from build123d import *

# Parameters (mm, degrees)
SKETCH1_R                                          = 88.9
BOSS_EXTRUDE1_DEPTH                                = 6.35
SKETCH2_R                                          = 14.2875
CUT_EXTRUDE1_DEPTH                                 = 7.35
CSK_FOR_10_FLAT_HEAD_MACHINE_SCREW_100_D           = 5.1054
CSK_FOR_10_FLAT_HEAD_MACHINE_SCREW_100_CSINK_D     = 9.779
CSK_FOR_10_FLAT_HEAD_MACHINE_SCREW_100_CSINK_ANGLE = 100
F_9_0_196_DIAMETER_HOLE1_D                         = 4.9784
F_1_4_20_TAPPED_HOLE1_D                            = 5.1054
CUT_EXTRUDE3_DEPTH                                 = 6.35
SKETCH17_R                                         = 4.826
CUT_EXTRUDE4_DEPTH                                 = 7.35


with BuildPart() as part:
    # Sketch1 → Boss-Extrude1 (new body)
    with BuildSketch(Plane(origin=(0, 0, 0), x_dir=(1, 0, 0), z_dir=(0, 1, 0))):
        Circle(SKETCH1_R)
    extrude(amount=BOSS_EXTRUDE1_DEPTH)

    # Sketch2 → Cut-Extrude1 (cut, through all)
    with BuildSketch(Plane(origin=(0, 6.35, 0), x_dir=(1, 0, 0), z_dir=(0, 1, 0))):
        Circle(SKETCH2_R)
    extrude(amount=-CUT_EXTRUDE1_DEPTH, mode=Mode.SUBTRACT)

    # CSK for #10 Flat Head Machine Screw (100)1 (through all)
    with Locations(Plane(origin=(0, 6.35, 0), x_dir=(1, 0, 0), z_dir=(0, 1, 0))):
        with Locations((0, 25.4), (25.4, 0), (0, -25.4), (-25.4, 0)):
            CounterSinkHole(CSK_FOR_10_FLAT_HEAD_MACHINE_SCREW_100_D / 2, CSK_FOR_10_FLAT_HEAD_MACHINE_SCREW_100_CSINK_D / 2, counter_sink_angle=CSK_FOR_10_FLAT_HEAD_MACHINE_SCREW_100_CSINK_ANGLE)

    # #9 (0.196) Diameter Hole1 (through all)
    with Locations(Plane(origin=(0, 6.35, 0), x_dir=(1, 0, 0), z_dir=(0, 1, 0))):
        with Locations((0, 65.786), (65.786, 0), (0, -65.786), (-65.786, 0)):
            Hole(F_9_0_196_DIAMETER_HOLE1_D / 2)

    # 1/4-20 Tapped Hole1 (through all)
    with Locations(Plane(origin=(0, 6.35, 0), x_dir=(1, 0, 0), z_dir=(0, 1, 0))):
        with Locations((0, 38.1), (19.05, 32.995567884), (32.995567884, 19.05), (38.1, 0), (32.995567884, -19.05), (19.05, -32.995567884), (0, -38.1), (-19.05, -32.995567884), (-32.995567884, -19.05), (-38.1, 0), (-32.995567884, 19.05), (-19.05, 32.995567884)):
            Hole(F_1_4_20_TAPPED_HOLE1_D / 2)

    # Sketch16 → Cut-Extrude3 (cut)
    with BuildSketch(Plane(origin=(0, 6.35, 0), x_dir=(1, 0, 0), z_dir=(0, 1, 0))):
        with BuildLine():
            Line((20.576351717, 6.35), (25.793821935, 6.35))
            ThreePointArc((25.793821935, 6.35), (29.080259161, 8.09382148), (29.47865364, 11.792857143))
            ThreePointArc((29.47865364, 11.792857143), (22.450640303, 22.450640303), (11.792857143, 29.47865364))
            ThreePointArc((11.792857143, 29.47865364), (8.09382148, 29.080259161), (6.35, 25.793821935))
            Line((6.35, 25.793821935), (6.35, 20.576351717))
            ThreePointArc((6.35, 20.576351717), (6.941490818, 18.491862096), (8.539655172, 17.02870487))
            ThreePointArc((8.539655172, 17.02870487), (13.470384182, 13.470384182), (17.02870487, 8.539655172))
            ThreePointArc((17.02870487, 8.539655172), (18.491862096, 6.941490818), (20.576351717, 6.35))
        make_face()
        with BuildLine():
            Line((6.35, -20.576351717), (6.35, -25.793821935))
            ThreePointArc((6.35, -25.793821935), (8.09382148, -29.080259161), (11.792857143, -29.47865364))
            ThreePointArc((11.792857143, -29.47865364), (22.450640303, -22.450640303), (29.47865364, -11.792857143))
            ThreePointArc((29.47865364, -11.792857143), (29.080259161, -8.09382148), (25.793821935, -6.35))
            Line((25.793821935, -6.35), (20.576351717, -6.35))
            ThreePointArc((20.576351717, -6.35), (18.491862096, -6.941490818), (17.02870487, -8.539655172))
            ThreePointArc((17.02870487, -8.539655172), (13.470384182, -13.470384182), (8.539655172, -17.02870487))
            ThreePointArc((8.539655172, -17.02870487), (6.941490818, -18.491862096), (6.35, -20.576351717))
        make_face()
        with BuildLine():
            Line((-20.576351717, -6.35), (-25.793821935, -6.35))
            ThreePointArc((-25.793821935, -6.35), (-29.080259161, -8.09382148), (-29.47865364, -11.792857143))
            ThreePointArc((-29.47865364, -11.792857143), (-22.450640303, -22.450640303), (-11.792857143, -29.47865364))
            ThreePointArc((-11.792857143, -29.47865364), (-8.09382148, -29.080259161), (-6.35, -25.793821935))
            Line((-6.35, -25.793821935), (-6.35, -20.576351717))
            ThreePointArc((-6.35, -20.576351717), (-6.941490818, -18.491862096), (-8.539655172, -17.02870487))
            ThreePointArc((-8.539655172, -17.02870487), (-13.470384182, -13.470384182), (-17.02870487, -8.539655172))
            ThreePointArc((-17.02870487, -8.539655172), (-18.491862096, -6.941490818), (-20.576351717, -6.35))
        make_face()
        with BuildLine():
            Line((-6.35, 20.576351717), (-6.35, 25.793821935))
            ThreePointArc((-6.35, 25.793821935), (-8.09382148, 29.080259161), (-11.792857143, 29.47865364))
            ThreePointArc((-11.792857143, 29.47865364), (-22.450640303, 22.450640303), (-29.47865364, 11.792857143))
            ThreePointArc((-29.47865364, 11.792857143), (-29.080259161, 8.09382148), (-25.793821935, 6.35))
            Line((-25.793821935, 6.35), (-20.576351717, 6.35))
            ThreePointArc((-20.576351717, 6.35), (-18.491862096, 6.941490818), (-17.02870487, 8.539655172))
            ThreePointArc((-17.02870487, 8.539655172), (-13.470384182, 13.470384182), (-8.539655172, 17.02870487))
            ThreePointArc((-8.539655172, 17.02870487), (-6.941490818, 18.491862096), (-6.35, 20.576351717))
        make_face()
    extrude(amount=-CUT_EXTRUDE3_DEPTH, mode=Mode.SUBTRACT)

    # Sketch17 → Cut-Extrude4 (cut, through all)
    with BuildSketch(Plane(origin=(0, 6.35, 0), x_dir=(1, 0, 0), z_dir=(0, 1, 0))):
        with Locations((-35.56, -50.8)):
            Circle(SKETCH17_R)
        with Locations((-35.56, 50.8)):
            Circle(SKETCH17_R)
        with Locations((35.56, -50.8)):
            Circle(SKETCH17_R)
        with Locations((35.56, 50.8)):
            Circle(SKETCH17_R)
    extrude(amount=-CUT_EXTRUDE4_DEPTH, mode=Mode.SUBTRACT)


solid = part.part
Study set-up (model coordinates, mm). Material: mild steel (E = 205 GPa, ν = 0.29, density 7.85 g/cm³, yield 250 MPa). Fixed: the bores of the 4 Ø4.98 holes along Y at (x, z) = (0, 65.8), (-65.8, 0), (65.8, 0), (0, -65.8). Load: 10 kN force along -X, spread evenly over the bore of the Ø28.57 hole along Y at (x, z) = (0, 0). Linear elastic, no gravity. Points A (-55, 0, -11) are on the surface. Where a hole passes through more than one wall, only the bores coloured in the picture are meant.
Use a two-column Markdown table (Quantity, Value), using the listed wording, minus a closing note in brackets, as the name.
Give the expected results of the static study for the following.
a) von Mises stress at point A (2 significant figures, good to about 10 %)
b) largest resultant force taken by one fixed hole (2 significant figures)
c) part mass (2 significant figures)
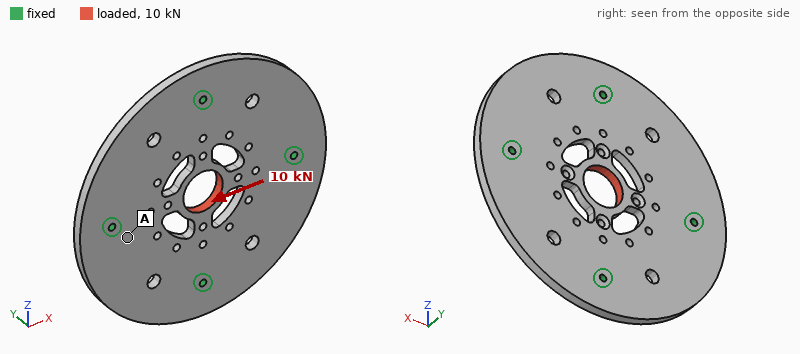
| Quantity | Value |
|---|---|
| von Mises stress at point A | 13 MPa |
| largest resultant force taken by one fixed hole | 3.2 kN |
| part mass | 1.1 kg |
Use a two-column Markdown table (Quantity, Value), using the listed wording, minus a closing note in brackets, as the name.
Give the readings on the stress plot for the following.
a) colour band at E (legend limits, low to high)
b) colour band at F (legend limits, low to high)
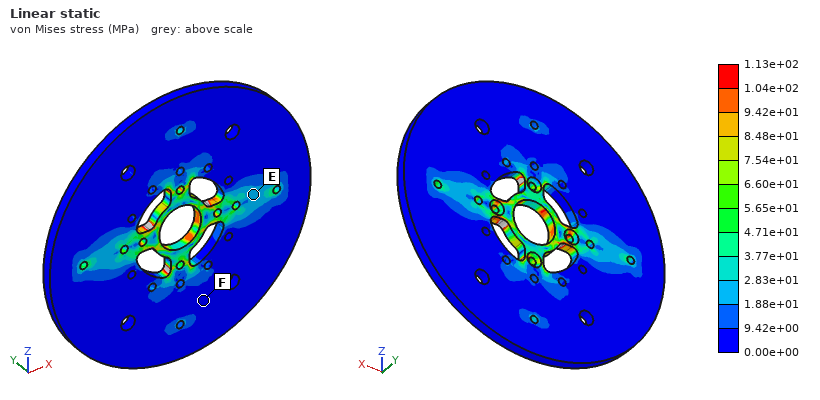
| Quantity | Value |
|---|---|
| colour band at E | 1.88e+01 to 2.83e+01 MPa |
| colour band at F | 0.00e+00 to 9.42e+00 MPa |
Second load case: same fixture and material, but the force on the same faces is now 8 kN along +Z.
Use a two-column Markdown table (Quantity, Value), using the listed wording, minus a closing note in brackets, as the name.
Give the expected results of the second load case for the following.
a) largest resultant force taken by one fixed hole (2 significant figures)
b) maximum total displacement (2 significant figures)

| Quantity | Value |
|---|---|
| largest resultant force taken by one fixed hole | 2.6 kN |
| maximum total displacement | 15 µm |
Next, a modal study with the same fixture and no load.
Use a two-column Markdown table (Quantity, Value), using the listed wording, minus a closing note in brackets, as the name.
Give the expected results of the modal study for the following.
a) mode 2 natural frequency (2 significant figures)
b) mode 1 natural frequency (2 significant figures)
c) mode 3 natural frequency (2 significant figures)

| Quantity | Value |
|---|---|
| mode 2 natural frequency | 2300 Hz |
| mode 1 natural frequency | 2000 Hz |
| mode 3 natural frequency | 2300 Hz |
